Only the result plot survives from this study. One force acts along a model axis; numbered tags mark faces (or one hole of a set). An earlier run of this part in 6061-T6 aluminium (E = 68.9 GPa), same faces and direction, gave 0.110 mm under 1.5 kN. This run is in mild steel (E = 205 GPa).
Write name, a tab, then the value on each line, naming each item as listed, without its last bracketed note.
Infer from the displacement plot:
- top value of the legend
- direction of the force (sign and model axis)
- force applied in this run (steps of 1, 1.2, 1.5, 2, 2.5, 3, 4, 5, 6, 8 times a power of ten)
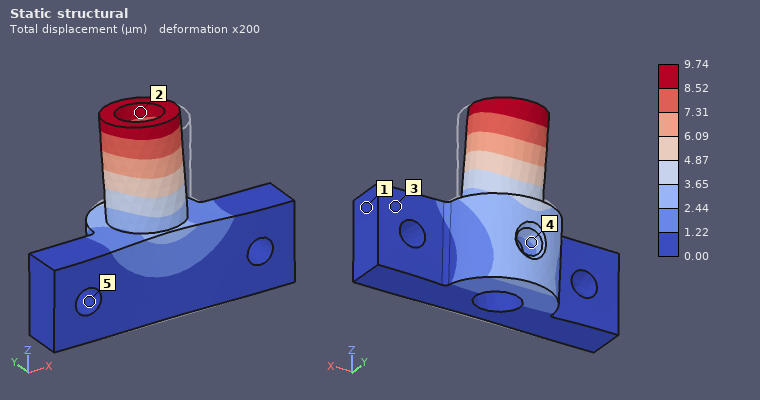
top value of the legend	9.74 µm
direction of the force	+Y
force applied in this run	400 N
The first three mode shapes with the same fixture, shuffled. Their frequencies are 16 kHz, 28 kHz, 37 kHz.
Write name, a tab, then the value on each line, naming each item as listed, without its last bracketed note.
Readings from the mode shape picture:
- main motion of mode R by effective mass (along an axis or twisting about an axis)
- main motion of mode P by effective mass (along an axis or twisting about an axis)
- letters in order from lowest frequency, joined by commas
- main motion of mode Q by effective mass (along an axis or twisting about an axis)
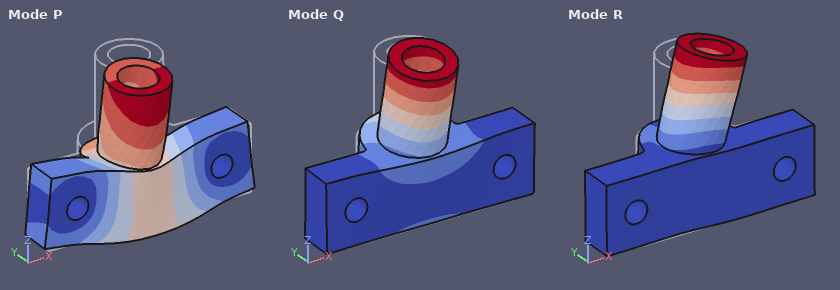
main motion of mode R by effective mass	along X
main motion of mode P by effective mass	along Z
letters in order from lowest frequency, joined by commas	Q, R, P
main motion of mode Q by effective mass	along Y
